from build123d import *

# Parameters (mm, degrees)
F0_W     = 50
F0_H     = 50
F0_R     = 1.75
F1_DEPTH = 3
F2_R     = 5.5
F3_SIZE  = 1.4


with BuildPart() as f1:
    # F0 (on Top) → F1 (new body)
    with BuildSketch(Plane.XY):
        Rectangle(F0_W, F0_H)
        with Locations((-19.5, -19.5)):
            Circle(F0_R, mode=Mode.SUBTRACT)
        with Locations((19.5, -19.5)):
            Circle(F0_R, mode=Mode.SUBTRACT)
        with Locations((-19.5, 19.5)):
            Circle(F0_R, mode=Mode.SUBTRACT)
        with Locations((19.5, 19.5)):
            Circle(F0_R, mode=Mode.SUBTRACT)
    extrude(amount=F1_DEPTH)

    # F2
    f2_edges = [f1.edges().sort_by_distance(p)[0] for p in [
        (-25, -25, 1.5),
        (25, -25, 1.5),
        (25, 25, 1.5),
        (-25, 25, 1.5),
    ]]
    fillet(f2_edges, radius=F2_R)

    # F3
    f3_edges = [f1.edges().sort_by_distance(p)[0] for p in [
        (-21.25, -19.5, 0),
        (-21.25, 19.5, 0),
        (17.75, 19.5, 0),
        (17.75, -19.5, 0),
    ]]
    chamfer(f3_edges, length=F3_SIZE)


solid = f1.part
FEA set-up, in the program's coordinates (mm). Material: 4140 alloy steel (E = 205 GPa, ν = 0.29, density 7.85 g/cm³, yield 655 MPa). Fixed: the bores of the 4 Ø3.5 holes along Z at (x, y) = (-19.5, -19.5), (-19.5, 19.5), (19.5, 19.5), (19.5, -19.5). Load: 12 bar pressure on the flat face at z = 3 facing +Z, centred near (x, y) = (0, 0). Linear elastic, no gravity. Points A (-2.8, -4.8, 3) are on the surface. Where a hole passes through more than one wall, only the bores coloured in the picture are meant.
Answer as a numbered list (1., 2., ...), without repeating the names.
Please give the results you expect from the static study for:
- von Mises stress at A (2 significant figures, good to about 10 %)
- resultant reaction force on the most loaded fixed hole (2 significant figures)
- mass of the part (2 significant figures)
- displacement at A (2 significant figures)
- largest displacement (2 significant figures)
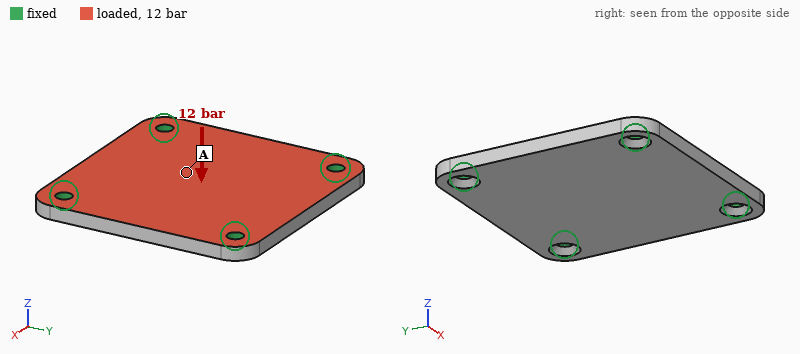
1. 60 MPa
2. 910 N
3. 57 g
4. 46 µm
5. 48 µm
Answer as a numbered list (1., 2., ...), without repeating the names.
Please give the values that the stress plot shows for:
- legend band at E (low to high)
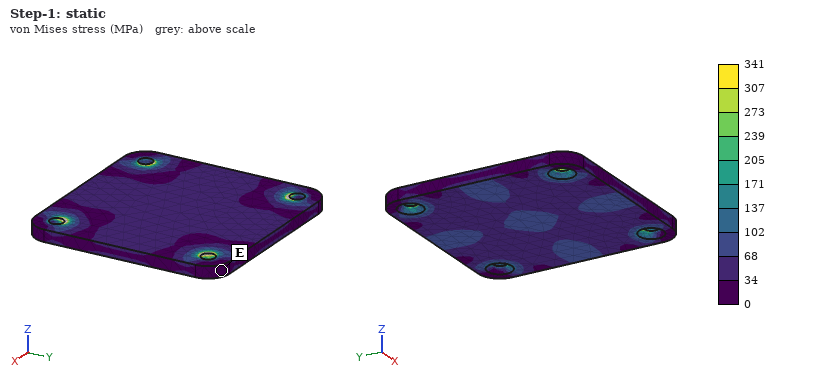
1. 0 to 34 MPa
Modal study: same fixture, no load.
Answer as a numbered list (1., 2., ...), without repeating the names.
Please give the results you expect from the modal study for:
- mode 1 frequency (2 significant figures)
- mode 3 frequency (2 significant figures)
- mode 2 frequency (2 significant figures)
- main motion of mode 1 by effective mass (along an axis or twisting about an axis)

1. 6300 Hz
2. 10 kHz
3. 10 kHz
4. along Z
